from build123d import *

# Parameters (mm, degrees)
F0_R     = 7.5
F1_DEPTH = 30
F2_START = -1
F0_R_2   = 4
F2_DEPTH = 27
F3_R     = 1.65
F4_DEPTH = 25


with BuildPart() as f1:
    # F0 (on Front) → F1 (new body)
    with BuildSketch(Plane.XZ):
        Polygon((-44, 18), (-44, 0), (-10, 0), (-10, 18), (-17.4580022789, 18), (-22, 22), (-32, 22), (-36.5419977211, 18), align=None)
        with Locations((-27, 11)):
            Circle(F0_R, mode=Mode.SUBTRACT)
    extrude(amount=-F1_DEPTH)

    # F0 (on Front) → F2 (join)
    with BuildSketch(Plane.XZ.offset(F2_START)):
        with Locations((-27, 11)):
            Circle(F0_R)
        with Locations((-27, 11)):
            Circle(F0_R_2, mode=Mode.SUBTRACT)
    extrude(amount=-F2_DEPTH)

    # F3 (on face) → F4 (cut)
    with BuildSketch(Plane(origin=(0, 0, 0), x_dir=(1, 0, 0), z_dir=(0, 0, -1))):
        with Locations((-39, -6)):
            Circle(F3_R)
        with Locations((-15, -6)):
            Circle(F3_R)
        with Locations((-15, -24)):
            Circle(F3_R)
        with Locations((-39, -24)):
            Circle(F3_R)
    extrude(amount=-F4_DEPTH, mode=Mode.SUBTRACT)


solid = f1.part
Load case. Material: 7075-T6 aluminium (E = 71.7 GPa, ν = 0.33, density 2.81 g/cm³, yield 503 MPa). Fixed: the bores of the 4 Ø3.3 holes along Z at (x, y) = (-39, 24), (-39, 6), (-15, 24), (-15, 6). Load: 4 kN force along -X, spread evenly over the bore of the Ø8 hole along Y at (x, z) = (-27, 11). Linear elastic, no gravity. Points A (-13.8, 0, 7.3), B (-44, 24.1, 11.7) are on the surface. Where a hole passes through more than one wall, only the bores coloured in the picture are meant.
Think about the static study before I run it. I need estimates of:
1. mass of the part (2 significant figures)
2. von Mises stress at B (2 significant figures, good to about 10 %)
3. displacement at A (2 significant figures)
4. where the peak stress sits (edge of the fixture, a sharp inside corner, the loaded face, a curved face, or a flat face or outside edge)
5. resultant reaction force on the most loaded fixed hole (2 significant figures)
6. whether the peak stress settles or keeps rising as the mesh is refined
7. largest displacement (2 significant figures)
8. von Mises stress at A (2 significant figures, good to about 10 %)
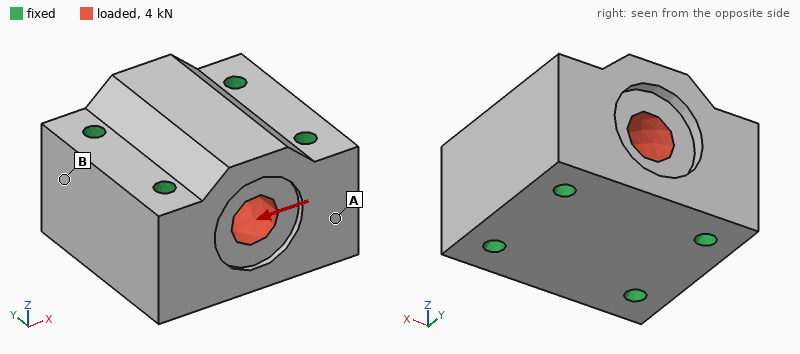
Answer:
49 g
2.6 MPa
0.21 µm
edge of the fixture
1.0 kN
keeps rising
1.1 µm
1.4 MPa
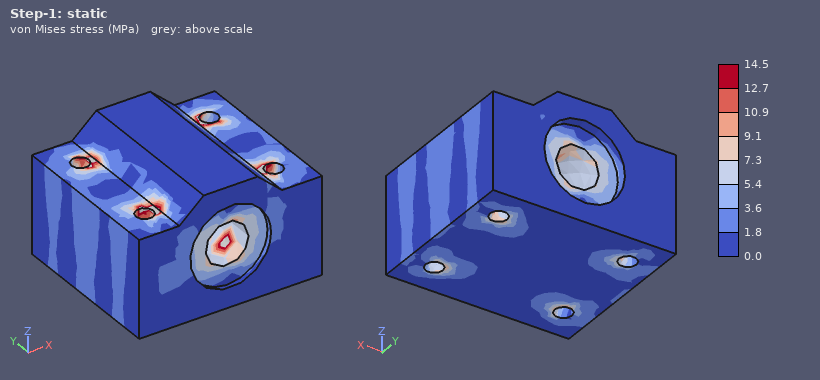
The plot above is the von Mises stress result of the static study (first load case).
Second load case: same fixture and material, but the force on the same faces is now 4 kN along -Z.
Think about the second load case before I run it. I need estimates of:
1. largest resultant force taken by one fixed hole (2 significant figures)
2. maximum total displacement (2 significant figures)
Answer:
1.0 kN
2.1 µm
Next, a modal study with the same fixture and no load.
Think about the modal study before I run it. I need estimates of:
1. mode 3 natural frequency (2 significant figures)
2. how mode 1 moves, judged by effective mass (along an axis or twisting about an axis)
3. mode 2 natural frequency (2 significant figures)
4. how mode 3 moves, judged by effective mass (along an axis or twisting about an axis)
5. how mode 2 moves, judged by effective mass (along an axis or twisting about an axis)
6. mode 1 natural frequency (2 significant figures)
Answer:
61 kHz
along Y
54 kHz
along Y
along Z
51 kHz
